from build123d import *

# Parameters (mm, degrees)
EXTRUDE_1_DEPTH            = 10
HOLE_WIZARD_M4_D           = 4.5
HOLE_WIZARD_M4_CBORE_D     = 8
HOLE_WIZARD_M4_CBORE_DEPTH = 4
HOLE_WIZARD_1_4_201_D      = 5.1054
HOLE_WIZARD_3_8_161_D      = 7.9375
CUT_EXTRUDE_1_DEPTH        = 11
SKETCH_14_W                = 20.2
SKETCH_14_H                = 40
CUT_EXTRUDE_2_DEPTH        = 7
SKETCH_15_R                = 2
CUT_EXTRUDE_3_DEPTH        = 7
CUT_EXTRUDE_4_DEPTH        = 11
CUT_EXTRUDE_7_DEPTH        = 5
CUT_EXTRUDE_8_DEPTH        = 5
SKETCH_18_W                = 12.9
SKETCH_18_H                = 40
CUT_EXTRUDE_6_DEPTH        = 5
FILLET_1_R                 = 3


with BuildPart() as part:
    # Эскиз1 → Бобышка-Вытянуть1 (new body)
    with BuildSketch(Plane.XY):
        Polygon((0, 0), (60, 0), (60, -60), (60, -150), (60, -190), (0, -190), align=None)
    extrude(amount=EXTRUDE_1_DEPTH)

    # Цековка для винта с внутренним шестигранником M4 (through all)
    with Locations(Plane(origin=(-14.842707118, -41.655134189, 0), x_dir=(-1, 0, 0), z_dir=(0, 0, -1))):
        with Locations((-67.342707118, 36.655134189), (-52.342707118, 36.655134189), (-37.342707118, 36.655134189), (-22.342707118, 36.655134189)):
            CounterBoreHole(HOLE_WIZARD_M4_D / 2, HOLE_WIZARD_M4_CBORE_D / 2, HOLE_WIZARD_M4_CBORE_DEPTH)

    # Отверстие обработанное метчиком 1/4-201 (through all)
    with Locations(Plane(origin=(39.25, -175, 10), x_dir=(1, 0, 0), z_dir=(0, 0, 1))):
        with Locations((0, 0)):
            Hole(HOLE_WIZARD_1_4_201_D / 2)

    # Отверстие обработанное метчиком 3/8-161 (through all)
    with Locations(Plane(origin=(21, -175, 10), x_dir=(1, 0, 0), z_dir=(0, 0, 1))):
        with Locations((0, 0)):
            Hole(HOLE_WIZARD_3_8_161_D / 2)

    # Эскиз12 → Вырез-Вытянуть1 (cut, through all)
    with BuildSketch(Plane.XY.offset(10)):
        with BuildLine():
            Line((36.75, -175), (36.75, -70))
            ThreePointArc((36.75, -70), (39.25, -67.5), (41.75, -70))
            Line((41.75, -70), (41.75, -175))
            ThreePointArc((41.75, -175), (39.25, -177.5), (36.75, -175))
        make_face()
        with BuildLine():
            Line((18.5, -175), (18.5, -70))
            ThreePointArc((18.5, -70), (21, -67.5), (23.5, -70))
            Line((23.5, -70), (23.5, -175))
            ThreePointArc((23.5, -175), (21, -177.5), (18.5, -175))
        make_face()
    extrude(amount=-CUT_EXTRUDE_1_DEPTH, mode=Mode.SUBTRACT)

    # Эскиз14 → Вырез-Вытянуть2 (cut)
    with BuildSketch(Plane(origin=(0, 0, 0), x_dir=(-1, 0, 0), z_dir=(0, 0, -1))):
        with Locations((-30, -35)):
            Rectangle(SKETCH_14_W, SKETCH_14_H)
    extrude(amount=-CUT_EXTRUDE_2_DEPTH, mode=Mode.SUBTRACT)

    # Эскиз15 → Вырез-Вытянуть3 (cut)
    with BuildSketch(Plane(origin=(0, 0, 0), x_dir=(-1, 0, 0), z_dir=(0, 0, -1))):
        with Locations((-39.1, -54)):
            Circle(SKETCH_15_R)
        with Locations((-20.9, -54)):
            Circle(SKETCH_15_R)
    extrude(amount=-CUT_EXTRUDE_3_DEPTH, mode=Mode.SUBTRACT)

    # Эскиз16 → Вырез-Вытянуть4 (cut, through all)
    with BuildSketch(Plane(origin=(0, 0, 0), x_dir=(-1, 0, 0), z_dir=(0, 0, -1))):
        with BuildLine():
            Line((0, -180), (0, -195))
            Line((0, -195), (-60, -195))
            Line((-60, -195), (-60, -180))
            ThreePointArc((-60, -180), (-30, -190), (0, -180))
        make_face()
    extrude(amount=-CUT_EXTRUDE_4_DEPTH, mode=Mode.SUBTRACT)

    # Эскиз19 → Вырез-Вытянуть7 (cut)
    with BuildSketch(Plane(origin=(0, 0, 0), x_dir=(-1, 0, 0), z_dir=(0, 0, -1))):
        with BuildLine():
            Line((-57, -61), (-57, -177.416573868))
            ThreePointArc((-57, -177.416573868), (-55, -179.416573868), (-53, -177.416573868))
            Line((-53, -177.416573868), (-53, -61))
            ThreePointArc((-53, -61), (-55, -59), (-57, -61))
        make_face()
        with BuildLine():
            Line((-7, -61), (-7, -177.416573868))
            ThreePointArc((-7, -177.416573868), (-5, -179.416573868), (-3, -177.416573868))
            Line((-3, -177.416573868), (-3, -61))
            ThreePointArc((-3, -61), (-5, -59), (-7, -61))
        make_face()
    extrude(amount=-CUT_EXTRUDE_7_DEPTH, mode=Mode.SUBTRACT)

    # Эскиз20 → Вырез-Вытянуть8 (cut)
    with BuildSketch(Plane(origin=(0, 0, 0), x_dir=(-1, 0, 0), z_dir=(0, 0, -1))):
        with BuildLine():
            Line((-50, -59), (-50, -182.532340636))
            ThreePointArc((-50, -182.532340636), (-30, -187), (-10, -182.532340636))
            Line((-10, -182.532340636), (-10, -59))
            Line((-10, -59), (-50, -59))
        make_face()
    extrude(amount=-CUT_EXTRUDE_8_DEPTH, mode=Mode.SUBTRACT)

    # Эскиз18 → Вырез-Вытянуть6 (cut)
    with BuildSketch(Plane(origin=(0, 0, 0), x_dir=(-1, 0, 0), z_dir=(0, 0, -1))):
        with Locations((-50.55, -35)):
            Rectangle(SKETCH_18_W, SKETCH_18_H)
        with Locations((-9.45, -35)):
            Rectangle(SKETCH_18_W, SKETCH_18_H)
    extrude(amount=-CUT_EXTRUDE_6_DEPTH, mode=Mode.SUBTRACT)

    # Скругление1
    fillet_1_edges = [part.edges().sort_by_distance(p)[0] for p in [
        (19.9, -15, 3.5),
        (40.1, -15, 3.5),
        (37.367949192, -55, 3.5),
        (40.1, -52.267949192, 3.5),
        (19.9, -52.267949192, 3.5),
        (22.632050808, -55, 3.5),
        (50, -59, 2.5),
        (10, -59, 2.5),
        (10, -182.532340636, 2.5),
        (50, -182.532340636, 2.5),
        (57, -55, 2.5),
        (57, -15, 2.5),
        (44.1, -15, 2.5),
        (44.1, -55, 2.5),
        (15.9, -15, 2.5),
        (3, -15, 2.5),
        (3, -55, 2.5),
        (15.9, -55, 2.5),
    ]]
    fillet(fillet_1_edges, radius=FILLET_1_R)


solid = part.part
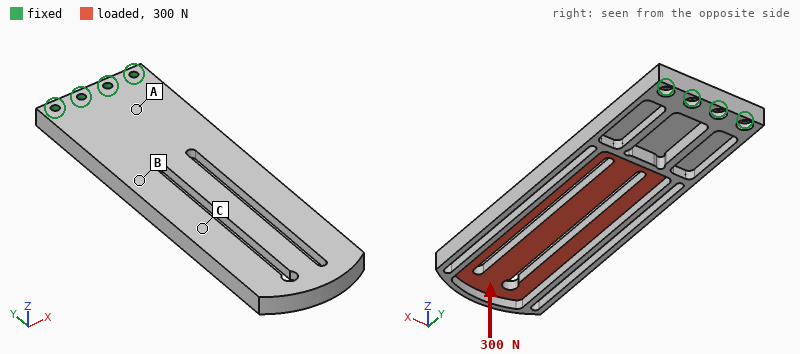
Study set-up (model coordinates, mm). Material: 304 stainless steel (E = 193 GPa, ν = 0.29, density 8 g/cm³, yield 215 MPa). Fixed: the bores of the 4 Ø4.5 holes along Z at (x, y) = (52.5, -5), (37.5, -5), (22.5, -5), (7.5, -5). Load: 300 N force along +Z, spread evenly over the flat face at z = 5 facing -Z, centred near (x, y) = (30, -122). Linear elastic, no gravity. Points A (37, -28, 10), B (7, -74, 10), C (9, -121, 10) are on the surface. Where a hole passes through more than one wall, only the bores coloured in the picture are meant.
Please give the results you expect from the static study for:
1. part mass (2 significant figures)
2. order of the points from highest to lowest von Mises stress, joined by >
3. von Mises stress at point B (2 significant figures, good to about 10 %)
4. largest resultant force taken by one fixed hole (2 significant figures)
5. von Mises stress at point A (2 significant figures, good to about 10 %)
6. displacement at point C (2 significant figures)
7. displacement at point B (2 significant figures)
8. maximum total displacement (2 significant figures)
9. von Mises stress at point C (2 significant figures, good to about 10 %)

520 g
A > B > C
28 MPa
280 N
42 MPa
0.39 mm
0.16 mm
0.79 mm
10 MPa
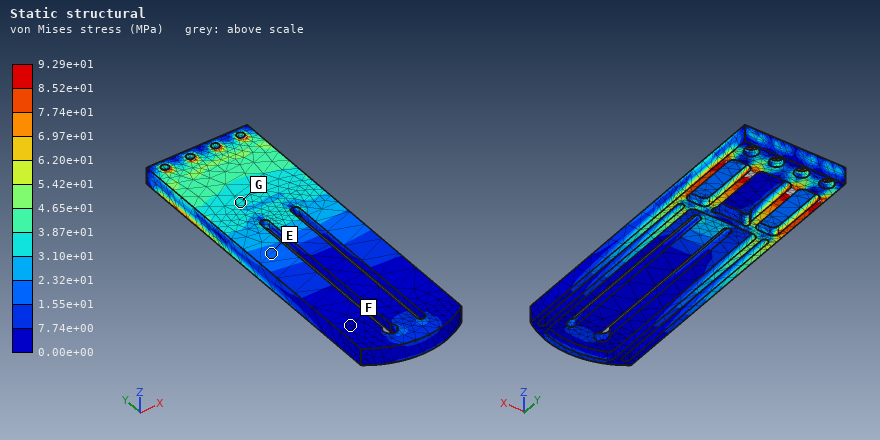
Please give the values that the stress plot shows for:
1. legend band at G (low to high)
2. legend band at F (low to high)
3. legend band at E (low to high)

3.10e+01 to 3.87e+01 MPa
0.00e+00 to 7.74e+00 MPa
1.55e+01 to 2.32e+01 MPa
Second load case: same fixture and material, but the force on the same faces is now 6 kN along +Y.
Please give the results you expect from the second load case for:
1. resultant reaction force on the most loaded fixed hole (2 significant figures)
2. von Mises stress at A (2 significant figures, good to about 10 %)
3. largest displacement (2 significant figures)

1.8 kN
6.3 MPa
0.37 mm
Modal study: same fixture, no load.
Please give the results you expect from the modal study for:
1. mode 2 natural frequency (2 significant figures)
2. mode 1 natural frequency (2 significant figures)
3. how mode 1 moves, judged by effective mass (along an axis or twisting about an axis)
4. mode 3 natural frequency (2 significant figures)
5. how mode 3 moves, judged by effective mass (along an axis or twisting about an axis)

680 Hz
210 Hz
along Z
970 Hz
along X
